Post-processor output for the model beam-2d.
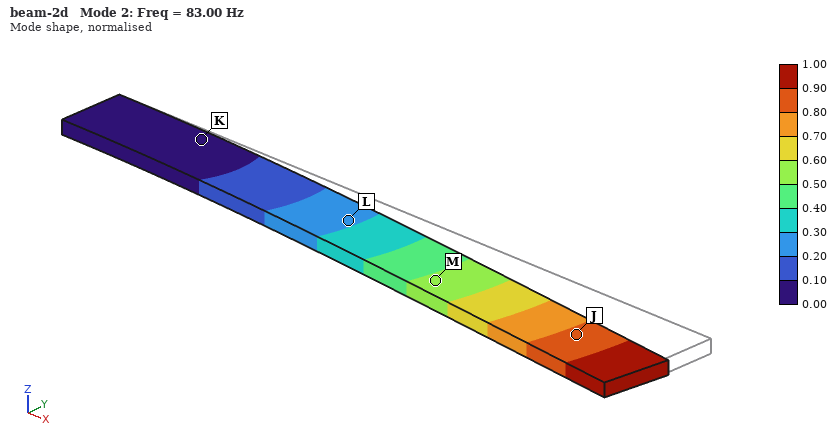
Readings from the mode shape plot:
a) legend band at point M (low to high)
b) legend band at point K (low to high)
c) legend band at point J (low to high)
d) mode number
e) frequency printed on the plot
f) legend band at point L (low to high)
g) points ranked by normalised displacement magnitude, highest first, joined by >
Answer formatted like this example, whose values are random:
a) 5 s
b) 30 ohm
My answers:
a) 0.50 to 0.60
b) 0.00 to 0.10
c) 0.80 to 0.90
d) 2
e) 83.00 Hz
f) 0.20 to 0.30
g) J > M > L > K
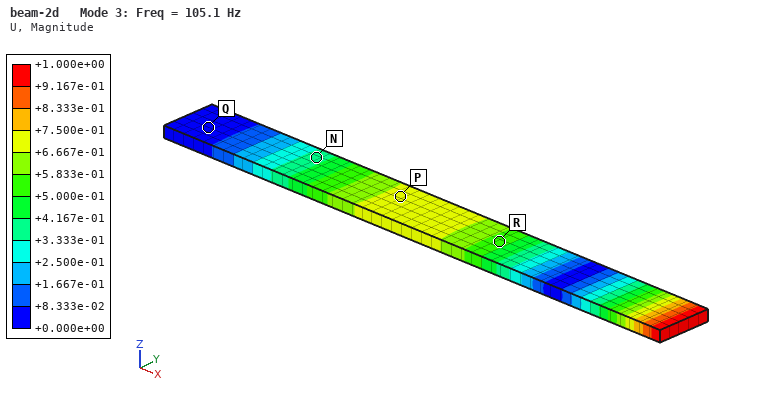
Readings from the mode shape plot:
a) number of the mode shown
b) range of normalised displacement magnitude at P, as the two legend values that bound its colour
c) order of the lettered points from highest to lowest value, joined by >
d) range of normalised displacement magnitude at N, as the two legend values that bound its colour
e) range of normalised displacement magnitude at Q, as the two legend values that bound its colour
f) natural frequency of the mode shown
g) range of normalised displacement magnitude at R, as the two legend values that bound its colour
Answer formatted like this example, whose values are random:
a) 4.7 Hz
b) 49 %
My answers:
a) 3
b) +6.667e-01 to +7.500e-01
c) P > R > N > Q
d) +3.333e-01 to +4.167e-01
e) +0.000e+00 to +8.333e-02
f) 105.1 Hz
g) +5.000e-01 to +5.833e-01
